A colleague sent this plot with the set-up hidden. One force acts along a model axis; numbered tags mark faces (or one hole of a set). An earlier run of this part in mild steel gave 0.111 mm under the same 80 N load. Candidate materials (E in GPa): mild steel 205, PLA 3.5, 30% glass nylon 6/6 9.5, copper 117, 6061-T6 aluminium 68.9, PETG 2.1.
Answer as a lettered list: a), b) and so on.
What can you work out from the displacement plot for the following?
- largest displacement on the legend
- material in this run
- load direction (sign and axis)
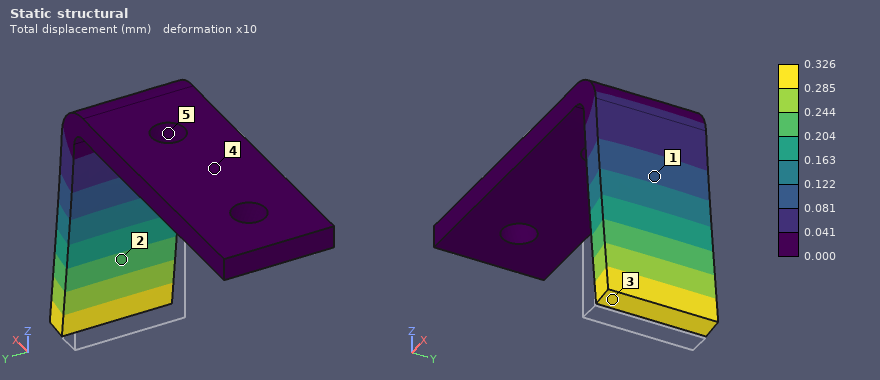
a) 0.326 mm
b) 6061-T6 aluminium
c) +X
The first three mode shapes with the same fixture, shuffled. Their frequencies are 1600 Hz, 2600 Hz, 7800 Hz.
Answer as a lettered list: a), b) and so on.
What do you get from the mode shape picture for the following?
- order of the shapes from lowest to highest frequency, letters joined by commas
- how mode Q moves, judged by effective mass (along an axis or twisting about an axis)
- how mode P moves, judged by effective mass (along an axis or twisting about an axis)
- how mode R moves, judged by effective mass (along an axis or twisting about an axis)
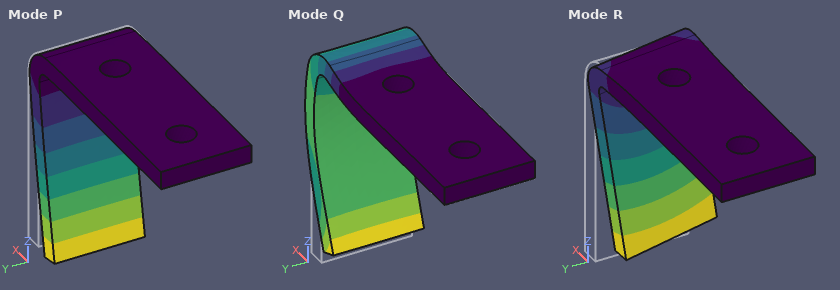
a) P, R, Q
b) along Z
c) along X
d) along Y
